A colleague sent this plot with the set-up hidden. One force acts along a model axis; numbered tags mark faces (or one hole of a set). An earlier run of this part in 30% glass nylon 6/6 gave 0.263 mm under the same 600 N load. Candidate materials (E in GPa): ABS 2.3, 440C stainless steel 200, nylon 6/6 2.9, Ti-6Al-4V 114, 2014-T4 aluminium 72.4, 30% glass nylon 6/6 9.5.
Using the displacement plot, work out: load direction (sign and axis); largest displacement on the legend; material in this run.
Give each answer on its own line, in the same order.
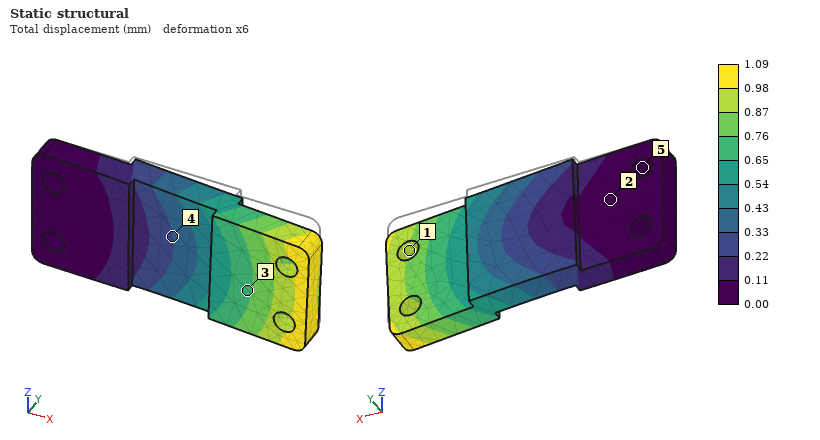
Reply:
-Z
1.09 mm
ABS
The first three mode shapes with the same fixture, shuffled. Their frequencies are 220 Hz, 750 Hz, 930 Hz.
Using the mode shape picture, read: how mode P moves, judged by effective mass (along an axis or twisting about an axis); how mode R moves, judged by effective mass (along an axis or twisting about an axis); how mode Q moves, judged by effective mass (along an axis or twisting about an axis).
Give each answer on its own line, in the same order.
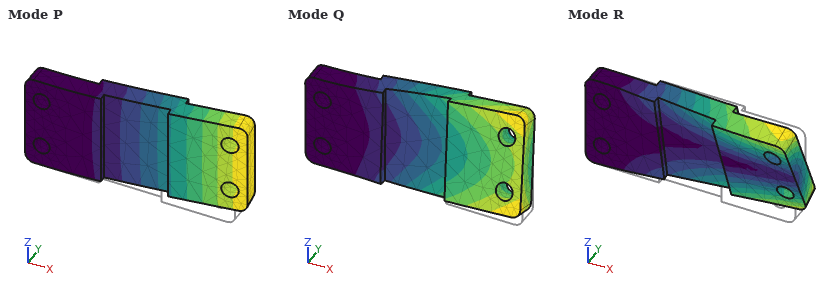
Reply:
along Y
along Z
along Z
